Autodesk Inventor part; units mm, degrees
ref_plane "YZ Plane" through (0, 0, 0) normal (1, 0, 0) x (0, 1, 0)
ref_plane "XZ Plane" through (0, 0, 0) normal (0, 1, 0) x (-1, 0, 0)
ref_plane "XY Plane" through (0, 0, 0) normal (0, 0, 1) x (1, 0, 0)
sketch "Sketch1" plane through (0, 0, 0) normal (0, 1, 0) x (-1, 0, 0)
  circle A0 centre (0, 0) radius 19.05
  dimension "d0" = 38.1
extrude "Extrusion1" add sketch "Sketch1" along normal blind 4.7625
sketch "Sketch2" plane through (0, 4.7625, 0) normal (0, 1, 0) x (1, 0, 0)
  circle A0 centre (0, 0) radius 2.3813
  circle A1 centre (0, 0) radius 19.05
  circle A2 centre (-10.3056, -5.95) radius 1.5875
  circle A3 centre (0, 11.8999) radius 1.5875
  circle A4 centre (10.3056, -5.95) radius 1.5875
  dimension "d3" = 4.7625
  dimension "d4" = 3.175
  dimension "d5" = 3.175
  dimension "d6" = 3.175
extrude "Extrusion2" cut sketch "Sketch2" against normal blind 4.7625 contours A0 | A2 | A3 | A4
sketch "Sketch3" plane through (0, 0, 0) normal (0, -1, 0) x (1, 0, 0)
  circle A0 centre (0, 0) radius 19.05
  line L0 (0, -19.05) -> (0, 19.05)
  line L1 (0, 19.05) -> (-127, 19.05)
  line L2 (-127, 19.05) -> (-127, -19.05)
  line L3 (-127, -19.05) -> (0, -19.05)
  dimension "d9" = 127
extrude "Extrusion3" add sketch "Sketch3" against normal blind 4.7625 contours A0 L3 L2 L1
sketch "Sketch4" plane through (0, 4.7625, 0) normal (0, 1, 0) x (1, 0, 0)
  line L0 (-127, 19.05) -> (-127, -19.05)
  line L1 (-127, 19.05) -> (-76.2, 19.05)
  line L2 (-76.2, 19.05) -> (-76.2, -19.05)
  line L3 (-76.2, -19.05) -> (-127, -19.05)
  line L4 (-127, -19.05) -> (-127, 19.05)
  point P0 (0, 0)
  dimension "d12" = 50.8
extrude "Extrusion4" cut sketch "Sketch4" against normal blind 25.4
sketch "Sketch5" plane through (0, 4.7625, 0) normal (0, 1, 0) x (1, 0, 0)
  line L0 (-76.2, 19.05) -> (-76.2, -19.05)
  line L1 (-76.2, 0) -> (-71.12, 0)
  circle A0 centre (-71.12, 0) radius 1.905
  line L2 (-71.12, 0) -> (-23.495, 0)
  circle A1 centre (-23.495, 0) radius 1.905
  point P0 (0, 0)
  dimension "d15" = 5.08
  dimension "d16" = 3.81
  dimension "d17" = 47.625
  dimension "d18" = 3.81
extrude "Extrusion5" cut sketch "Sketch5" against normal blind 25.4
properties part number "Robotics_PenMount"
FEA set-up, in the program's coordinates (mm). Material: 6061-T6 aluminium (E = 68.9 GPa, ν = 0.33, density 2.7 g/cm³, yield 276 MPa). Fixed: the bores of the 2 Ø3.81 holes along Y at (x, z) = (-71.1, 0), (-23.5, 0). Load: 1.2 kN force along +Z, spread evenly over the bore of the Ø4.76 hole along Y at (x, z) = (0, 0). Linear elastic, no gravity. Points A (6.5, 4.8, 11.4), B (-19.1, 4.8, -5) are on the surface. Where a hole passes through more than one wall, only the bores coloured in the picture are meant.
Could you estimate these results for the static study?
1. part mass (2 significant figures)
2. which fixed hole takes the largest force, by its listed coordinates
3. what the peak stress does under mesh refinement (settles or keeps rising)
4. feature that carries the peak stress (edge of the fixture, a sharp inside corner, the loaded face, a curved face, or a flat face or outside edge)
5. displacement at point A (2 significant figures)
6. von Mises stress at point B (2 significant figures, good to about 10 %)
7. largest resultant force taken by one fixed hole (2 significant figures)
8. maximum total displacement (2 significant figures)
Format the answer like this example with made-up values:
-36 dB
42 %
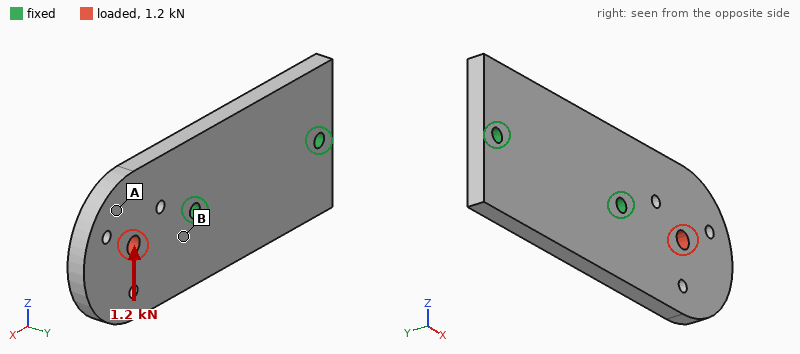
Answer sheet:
44 g
(-23.5, 0)
keeps rising
edge of the fixture
28 µm
20 MPa
1.7 kN
35 µm
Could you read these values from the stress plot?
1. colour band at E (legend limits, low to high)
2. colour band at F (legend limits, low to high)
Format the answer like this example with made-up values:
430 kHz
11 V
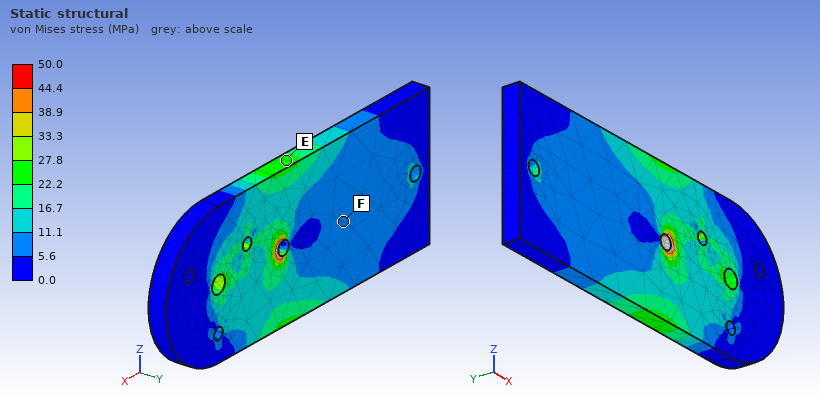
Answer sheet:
22.2 to 27.8 MPa
5.6 to 11.1 MPa
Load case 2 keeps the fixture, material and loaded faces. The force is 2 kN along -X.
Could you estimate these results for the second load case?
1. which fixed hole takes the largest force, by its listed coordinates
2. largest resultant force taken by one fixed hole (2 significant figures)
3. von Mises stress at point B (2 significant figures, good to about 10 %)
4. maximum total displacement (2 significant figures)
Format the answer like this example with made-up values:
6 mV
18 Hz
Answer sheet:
(-23.5, 0)
1.6 kN
14 MPa
9.3 µm
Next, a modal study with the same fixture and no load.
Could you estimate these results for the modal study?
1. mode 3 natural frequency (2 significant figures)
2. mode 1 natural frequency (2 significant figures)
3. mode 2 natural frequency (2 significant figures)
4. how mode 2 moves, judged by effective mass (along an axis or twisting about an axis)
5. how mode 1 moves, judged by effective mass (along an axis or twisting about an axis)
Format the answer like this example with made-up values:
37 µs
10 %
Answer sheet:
6700 Hz
2300 Hz
4700 Hz
twisting about X
along Y
